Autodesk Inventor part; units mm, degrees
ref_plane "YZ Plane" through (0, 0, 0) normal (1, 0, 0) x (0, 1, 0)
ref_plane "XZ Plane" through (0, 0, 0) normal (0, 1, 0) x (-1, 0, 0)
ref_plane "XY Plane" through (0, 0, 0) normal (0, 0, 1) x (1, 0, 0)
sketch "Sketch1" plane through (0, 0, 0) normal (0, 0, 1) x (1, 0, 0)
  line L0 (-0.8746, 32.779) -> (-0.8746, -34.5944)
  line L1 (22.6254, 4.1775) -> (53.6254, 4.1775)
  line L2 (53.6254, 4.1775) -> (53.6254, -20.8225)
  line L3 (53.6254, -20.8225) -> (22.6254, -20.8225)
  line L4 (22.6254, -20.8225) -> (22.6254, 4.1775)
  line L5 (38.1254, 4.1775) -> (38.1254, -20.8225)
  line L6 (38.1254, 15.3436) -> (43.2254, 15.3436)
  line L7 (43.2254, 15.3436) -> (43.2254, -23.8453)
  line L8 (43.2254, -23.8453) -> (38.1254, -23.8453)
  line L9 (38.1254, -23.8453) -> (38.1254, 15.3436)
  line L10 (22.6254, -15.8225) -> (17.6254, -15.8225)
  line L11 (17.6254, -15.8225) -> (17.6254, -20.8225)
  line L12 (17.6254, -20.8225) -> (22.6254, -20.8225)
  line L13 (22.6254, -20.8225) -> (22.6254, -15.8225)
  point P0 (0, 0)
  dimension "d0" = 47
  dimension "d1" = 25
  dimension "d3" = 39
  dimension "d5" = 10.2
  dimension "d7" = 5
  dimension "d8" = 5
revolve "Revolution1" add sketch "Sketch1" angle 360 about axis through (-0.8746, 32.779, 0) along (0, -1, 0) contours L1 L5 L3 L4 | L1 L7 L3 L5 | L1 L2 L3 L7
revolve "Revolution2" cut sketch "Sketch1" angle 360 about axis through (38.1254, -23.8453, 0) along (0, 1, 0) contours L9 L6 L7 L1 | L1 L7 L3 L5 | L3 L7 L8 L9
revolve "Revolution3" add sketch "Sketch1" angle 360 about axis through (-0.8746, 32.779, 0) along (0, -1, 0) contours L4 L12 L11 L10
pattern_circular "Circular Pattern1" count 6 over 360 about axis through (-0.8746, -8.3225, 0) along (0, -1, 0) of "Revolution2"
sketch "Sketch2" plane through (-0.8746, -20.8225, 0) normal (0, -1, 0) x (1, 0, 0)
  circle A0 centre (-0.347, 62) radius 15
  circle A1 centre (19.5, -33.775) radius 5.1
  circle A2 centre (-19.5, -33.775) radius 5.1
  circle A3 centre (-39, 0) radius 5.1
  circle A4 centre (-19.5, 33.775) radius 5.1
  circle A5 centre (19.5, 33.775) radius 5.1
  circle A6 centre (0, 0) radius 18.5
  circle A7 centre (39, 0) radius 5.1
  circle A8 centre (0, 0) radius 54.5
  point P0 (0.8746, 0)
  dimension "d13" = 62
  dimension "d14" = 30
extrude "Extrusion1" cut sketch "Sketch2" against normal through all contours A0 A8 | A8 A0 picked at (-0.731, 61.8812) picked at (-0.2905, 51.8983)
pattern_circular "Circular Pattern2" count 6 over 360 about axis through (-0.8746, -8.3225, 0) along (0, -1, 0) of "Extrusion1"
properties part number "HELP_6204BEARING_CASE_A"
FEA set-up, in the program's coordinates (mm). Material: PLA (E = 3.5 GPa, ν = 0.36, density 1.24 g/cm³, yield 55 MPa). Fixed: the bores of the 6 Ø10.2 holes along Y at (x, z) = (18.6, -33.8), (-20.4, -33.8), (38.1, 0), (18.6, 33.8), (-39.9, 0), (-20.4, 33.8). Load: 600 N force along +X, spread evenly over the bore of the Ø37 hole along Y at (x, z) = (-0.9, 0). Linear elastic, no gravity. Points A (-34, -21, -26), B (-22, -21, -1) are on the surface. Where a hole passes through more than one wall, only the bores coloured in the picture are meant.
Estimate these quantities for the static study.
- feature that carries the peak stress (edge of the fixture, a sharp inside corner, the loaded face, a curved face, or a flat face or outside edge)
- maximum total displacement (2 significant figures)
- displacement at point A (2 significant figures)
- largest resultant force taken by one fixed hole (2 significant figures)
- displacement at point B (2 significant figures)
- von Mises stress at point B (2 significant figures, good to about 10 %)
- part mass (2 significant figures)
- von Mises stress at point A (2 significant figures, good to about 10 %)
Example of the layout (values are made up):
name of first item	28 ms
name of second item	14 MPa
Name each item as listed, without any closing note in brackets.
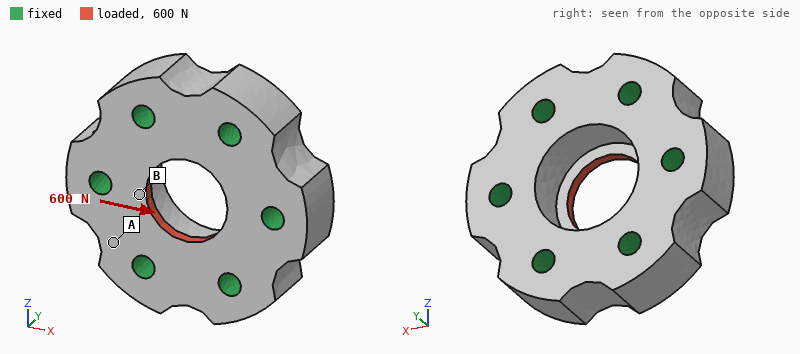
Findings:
feature that carries the peak stress	a sharp inside corner
maximum total displacement	6.5 µm
displacement at point A	1.2 µm
largest resultant force taken by one fixed hole	150 N
displacement at point B	5.0 µm
von Mises stress at point B	1.1 MPa
part mass	200 g
von Mises stress at point A	0.20 MPa
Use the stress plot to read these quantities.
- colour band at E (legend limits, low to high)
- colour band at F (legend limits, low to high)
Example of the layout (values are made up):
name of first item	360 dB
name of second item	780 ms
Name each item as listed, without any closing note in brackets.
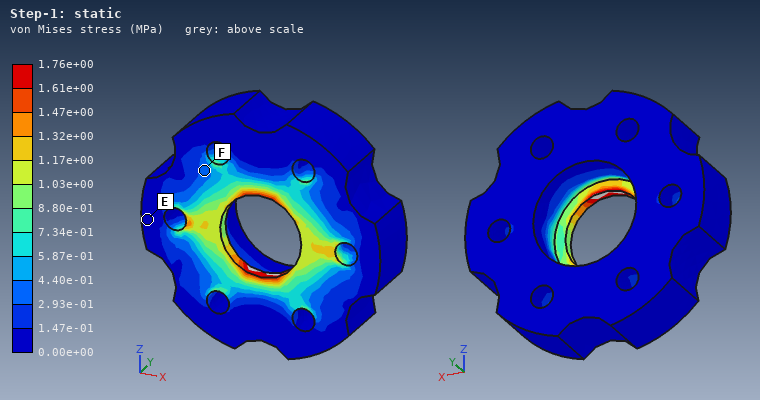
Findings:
colour band at E	0.00e+00 to 1.47e-01 MPa
colour band at F	2.93e-01 to 4.40e-01 MPa
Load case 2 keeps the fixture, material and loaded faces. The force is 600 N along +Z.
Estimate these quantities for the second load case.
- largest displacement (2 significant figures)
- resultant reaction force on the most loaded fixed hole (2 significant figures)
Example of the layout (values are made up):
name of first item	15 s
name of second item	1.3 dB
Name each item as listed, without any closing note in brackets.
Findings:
largest displacement	6.9 µm
resultant reaction force on the most loaded fixed hole	130 N
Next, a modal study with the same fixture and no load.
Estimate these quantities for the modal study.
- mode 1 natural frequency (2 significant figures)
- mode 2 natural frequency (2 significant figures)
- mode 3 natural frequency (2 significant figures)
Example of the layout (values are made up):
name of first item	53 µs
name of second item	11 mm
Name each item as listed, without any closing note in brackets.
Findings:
mode 1 natural frequency	11 kHz
mode 2 natural frequency	12 kHz
mode 3 natural frequency	12 kHz
